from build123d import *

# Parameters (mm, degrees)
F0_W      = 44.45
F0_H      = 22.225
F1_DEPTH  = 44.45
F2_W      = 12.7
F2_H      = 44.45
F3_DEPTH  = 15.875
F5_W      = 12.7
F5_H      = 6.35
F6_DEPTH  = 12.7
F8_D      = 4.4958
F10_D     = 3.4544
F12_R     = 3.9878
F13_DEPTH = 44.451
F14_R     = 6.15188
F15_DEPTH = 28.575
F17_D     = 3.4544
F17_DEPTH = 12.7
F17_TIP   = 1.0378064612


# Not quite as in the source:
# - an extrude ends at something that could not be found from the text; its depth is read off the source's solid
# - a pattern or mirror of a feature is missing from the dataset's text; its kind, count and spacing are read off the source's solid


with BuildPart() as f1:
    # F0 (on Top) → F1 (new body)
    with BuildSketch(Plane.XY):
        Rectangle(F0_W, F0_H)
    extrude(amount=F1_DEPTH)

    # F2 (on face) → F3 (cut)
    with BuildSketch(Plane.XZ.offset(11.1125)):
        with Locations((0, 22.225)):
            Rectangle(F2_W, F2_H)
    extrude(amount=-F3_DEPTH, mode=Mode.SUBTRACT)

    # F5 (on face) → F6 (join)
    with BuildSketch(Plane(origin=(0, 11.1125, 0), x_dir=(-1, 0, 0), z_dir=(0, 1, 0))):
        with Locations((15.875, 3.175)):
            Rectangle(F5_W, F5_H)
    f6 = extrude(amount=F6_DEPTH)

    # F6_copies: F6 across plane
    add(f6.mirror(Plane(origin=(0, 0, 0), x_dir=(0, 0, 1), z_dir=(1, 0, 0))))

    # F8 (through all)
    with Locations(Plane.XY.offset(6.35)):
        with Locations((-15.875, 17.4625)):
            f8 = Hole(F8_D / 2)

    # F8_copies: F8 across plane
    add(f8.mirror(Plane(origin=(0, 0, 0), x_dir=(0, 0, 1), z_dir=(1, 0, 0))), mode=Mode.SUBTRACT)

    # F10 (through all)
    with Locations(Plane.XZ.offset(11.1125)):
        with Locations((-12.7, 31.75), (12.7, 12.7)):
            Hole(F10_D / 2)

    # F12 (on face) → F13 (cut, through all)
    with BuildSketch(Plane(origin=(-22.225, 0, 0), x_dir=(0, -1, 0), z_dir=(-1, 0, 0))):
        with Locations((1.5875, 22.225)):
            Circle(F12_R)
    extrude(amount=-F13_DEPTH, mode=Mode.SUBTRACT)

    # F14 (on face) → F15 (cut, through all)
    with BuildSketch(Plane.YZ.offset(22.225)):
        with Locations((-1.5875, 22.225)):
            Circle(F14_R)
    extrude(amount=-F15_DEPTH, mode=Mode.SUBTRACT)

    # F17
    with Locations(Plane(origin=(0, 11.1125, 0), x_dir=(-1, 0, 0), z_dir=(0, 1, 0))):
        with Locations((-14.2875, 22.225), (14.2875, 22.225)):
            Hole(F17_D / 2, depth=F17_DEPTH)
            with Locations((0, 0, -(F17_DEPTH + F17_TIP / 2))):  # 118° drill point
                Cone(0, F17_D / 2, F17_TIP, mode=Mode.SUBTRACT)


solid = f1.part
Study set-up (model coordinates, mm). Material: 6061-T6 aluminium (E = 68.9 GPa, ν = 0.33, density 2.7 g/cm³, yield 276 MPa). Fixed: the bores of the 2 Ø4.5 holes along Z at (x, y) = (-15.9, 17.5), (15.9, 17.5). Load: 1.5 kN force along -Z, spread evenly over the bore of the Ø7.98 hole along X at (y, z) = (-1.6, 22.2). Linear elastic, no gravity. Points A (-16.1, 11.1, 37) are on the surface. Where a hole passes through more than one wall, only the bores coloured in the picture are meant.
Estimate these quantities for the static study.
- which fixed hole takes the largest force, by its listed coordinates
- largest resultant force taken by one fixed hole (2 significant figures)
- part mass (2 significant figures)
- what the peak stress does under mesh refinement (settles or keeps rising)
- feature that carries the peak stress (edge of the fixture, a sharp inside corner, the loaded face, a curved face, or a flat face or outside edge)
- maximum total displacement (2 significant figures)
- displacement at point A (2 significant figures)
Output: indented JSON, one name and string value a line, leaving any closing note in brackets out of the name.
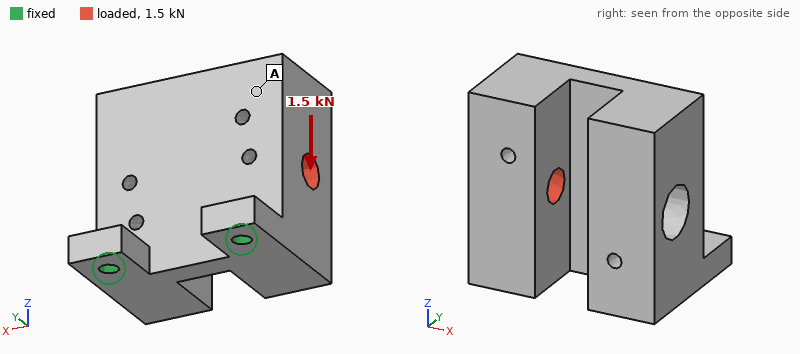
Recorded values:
{
  "which fixed hole takes the largest force, by its listed coordinates": "(-15.9, 17.5)",
  "largest resultant force taken by one fixed hole": "1.4 kN",
  "part mass": "91 g",
  "what the peak stress does under mesh refinement": "keeps rising",
  "feature that carries the peak stress": "edge of the fixture",
  "maximum total displacement": "0.26 mm",
  "displacement at point A": "0.18 mm"
}
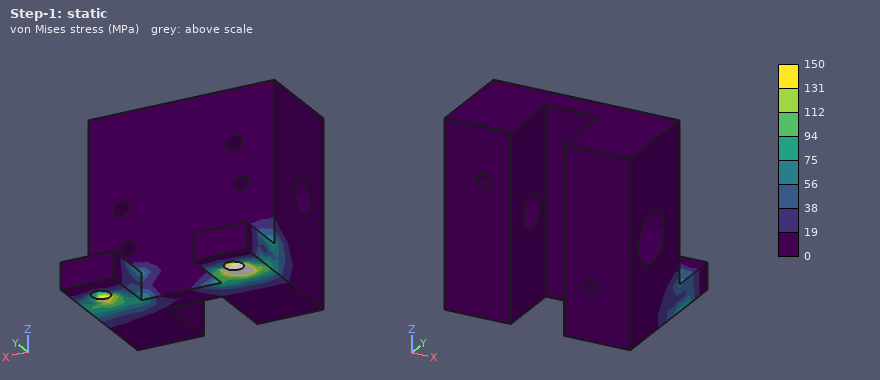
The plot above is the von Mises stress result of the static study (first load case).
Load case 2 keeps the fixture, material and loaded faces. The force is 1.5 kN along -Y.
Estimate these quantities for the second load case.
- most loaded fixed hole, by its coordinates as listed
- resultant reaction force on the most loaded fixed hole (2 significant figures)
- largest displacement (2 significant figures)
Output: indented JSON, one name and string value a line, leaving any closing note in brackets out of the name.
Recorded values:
{
  "most loaded fixed hole, by its coordinates as listed": "(-15.9, 17.5)",
  "resultant reaction force on the most loaded fixed hole": "1.3 kN",
  "largest displacement": "0.34 mm"
}
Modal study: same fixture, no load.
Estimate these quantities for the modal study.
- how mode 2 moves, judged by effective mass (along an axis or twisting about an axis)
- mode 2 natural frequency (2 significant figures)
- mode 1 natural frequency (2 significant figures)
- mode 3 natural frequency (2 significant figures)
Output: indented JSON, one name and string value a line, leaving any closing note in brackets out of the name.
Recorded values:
{
  "how mode 2 moves, judged by effective mass": "along X",
  "mode 2 natural frequency": "4400 Hz",
  "mode 1 natural frequency": "1300 Hz",
  "mode 3 natural frequency": "4700 Hz"
}
